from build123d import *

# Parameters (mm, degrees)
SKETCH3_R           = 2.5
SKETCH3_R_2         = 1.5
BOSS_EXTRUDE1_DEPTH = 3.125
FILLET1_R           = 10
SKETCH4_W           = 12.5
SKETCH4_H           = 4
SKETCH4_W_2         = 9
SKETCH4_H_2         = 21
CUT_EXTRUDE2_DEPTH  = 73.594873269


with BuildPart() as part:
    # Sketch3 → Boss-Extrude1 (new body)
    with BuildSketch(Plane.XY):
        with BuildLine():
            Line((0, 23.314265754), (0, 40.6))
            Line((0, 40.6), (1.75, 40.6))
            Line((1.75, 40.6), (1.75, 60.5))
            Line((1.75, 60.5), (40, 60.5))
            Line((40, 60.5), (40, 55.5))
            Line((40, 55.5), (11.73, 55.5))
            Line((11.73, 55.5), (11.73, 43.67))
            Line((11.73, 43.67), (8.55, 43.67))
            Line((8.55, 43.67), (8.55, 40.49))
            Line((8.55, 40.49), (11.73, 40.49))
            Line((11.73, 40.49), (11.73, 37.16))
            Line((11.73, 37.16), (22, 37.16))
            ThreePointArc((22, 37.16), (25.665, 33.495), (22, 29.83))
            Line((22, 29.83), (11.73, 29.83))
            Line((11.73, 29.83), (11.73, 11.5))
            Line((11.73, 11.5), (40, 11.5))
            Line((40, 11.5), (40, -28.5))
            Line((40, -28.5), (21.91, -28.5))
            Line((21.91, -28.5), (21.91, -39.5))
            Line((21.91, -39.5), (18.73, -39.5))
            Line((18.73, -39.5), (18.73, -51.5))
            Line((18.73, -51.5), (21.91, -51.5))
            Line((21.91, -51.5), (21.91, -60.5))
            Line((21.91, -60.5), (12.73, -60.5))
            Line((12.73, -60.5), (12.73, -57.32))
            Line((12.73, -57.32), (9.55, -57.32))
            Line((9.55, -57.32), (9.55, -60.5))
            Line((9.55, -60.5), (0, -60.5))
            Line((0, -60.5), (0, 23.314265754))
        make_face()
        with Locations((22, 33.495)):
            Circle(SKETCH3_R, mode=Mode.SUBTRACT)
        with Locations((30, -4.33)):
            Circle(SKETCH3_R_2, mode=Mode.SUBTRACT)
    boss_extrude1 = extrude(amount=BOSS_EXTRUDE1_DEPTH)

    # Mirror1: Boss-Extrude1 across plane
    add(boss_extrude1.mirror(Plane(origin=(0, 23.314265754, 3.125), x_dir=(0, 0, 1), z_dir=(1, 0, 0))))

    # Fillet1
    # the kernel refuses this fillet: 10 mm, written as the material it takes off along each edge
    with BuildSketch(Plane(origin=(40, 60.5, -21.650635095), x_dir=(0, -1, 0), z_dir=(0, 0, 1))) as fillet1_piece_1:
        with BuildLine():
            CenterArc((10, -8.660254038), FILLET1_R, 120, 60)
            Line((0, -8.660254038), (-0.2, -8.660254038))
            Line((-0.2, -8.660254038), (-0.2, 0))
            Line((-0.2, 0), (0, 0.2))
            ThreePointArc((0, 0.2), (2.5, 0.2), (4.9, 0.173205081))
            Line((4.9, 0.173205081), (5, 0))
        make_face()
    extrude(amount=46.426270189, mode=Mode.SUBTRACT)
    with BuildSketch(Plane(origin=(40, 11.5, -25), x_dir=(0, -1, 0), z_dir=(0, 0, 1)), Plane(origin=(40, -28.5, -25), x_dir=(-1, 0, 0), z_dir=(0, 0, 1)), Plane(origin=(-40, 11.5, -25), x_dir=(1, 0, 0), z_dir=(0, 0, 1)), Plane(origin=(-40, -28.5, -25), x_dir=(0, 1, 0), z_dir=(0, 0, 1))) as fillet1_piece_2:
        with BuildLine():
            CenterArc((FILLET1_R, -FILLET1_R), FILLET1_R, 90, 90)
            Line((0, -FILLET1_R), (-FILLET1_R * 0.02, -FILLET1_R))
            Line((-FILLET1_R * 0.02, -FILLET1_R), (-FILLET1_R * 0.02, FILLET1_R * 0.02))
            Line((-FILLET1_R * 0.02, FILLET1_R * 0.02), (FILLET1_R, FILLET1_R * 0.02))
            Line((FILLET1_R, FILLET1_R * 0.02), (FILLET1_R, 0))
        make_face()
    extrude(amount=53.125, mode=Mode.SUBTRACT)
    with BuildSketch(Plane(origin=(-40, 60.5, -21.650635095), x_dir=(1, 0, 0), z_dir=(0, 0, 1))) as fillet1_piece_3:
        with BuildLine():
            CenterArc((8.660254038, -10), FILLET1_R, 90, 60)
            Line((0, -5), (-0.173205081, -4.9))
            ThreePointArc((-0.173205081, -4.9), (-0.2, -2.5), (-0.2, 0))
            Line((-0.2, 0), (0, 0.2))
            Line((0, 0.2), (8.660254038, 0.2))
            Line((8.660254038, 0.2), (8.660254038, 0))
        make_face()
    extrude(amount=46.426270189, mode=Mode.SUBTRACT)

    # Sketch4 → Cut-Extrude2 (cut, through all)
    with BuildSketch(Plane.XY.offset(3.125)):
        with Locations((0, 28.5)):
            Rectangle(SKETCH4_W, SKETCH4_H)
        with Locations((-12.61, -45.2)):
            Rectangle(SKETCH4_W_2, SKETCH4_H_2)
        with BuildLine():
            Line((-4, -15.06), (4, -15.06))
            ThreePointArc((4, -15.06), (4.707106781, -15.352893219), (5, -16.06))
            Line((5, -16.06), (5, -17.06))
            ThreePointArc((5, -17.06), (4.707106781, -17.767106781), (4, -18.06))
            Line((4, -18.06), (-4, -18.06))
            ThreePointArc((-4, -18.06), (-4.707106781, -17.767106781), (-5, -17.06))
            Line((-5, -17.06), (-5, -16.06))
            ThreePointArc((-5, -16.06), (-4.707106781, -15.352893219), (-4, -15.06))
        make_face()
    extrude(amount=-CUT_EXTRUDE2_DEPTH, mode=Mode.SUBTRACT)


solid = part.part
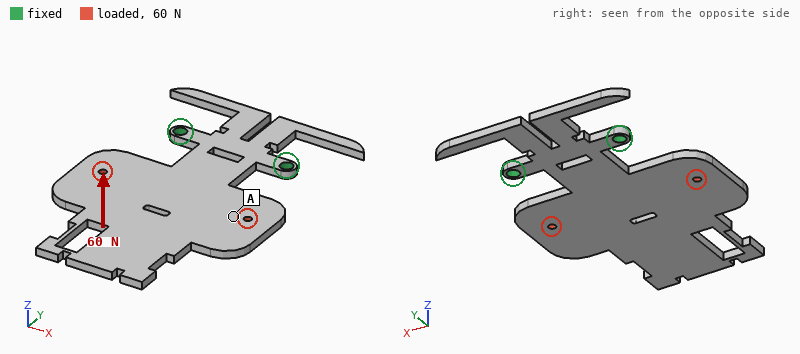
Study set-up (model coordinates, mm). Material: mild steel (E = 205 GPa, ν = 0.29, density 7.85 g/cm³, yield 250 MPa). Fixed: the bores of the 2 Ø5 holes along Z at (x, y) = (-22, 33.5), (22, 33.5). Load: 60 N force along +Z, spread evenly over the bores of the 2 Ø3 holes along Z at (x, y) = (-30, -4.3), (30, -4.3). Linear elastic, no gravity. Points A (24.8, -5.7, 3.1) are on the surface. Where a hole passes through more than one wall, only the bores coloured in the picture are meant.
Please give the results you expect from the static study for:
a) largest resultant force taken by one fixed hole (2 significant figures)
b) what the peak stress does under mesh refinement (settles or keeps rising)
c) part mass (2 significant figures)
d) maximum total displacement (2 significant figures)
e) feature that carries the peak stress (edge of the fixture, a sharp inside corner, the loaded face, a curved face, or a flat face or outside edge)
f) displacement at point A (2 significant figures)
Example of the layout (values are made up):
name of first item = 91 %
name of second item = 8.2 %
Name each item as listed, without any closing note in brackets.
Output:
largest resultant force taken by one fixed hole = 30 N
what the peak stress does under mesh refinement = keeps rising
part mass = 140 g
maximum total displacement = 0.58 mm
feature that carries the peak stress = a sharp inside corner
displacement at point A = 0.22 mm
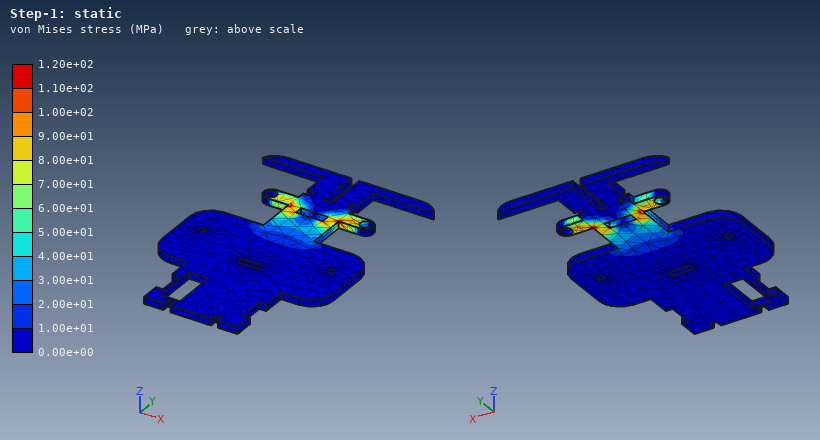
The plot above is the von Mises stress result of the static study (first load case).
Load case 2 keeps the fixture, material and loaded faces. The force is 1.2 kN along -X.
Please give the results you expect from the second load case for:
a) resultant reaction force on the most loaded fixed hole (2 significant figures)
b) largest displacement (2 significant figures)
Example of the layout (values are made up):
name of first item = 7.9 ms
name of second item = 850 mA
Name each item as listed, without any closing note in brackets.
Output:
resultant reaction force on the most loaded fixed hole = 1.5 kN
largest displacement = 0.20 mm
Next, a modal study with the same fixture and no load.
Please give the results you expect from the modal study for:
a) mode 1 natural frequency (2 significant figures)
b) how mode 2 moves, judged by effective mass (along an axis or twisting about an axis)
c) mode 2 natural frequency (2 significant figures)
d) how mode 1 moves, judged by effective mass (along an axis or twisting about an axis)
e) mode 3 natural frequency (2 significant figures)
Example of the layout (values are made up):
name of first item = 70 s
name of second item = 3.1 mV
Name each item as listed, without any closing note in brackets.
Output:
mode 1 natural frequency = 170 Hz
how mode 2 moves, judged by effective mass = twisting about Y
mode 2 natural frequency = 580 Hz
how mode 1 moves, judged by effective mass = along Z
mode 3 natural frequency = 1100 Hz
